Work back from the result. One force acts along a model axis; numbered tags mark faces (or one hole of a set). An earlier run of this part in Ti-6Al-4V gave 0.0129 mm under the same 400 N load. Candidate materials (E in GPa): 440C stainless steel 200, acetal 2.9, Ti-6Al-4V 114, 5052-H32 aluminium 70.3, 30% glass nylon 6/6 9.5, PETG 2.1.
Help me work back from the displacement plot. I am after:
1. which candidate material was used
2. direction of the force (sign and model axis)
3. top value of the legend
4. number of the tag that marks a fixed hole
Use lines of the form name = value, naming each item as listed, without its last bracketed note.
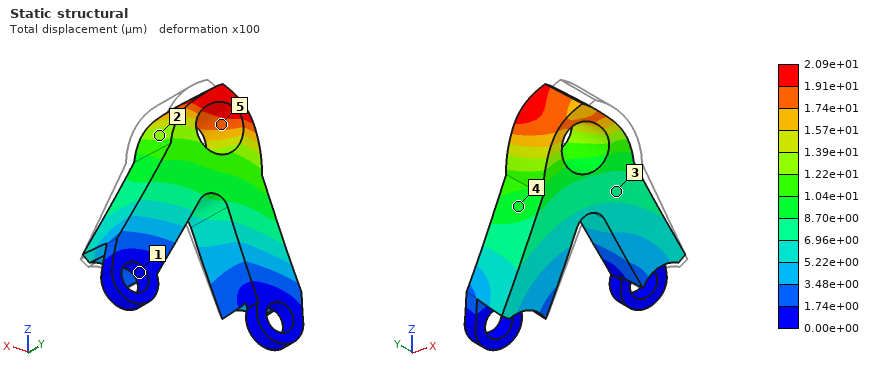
which candidate material was used = 5052-H32 aluminium
direction of the force = -X
top value of the legend = 2.09e+01 µm
number of the tag that marks a fixed hole = 1
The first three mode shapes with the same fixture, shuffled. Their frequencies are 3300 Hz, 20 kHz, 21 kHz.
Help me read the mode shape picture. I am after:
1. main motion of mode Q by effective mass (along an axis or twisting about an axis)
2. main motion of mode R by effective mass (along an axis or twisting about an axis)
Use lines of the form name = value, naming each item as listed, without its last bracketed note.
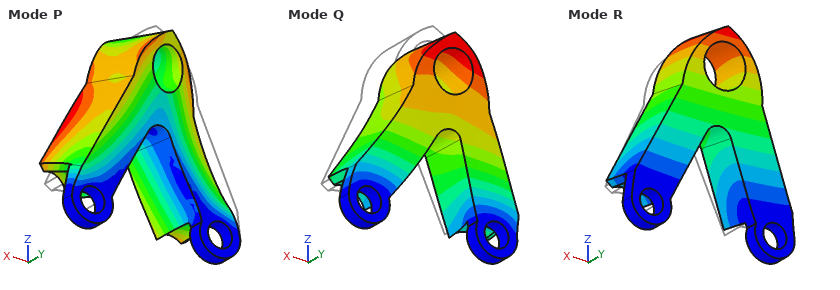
main motion of mode Q by effective mass = along X
main motion of mode R by effective mass = along Y
